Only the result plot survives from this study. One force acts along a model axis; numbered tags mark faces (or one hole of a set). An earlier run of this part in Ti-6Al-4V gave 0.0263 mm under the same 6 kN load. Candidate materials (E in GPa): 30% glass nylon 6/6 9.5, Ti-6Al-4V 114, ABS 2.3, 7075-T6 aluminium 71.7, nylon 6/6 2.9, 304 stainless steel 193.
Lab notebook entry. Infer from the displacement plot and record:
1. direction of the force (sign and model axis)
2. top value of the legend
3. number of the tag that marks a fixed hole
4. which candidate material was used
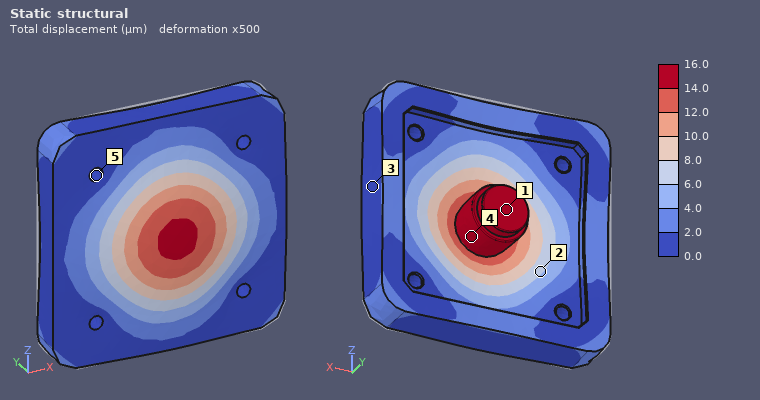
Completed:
-Y
16.0 µm
5
304 stainless steel
